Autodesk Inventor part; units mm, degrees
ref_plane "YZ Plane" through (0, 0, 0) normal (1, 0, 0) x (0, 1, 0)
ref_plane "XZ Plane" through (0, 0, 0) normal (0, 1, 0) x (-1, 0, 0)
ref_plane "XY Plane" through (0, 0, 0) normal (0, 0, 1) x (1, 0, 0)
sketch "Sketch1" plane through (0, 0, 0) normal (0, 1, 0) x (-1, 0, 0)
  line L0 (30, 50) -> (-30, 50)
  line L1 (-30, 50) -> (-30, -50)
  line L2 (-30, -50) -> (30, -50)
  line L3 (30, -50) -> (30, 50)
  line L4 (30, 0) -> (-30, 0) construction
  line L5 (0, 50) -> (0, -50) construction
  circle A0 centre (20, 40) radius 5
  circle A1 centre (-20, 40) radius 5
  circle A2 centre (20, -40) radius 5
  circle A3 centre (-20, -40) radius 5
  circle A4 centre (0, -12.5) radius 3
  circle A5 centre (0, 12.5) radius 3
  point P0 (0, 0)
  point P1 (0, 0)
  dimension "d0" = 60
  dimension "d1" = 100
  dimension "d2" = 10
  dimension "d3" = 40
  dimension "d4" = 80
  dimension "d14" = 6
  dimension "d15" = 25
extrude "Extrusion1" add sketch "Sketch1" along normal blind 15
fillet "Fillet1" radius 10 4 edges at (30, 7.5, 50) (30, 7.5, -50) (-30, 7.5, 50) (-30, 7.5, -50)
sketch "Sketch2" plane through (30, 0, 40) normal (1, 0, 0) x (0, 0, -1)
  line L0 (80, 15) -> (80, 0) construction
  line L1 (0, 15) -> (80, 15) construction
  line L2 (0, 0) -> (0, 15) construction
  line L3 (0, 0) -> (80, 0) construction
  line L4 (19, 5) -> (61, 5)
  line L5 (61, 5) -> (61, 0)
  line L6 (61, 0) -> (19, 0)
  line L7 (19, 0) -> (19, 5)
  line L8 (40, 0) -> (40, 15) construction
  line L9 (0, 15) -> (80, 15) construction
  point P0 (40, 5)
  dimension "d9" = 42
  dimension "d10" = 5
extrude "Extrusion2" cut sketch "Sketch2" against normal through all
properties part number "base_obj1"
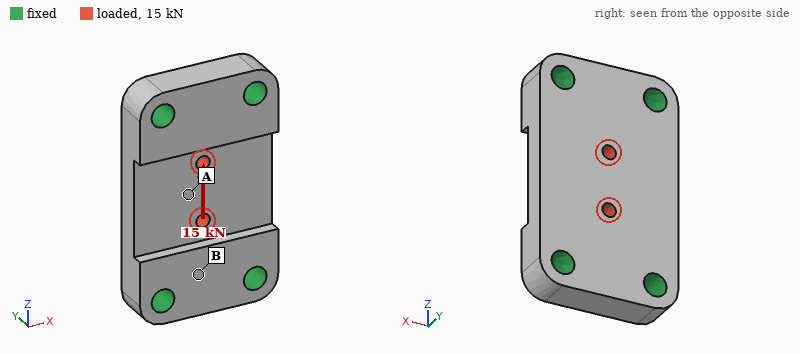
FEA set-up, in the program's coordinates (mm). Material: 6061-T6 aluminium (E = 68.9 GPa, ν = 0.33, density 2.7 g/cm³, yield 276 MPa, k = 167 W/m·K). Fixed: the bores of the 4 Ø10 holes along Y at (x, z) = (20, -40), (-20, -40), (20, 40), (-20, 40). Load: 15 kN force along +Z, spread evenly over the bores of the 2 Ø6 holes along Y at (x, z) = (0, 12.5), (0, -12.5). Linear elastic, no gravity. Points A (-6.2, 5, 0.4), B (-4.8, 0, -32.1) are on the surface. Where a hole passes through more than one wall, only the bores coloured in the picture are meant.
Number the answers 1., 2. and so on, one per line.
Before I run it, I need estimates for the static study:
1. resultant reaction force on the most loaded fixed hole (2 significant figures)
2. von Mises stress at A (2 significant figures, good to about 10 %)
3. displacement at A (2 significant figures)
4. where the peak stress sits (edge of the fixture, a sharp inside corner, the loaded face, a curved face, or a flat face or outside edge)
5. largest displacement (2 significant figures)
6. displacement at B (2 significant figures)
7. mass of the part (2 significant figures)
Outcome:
1. 4.0 kN
2. 20 MPa
3. 8.2 µm
4. the loaded face
5. 12 µm
6. 2.2 µm
7. 190 g
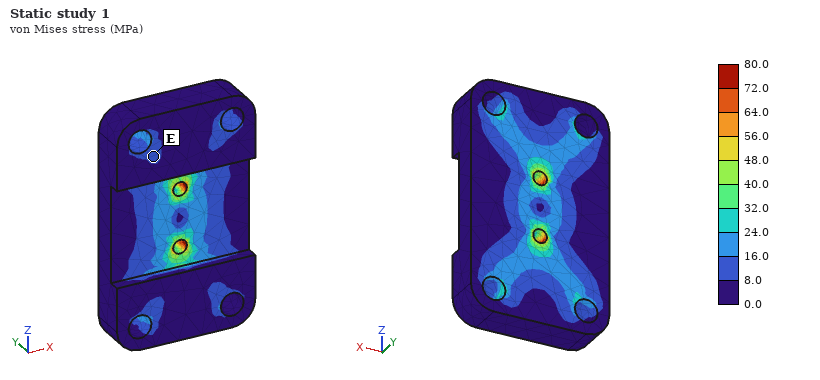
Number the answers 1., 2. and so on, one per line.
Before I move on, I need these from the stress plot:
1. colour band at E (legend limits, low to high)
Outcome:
1. 8.0 to 16.0 MPa
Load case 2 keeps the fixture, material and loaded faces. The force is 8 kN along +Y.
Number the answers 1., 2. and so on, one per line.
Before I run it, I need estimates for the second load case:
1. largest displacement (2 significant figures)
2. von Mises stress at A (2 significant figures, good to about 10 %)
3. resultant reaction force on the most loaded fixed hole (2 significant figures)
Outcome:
1. 39 µm
2. 28 MPa
3. 2.3 kN
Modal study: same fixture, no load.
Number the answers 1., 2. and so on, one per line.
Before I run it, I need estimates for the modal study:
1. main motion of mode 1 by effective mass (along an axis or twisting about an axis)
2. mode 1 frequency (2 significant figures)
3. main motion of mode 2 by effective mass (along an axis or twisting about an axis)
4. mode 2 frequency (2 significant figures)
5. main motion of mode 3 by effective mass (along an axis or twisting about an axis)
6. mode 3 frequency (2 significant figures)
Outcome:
1. along Y
2. 11 kHz
3. twisting about Z
4. 14 kHz
5. along X
6. 19 kHz
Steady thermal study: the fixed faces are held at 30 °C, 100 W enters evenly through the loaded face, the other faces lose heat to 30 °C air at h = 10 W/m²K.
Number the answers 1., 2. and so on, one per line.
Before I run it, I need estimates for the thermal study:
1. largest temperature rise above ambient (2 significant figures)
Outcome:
1. 19 K
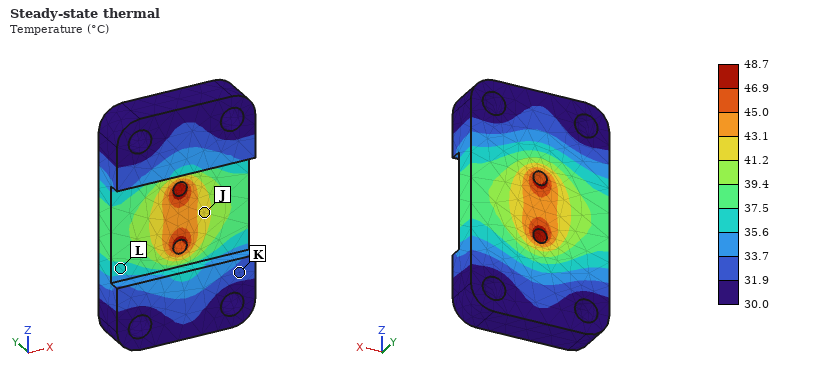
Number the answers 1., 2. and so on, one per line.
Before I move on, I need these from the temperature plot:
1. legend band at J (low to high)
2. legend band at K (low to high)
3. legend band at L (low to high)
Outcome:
1. 41.2 to 43.1 °C
2. 31.9 to 33.7 °C
3. 35.6 to 37.5 °C
